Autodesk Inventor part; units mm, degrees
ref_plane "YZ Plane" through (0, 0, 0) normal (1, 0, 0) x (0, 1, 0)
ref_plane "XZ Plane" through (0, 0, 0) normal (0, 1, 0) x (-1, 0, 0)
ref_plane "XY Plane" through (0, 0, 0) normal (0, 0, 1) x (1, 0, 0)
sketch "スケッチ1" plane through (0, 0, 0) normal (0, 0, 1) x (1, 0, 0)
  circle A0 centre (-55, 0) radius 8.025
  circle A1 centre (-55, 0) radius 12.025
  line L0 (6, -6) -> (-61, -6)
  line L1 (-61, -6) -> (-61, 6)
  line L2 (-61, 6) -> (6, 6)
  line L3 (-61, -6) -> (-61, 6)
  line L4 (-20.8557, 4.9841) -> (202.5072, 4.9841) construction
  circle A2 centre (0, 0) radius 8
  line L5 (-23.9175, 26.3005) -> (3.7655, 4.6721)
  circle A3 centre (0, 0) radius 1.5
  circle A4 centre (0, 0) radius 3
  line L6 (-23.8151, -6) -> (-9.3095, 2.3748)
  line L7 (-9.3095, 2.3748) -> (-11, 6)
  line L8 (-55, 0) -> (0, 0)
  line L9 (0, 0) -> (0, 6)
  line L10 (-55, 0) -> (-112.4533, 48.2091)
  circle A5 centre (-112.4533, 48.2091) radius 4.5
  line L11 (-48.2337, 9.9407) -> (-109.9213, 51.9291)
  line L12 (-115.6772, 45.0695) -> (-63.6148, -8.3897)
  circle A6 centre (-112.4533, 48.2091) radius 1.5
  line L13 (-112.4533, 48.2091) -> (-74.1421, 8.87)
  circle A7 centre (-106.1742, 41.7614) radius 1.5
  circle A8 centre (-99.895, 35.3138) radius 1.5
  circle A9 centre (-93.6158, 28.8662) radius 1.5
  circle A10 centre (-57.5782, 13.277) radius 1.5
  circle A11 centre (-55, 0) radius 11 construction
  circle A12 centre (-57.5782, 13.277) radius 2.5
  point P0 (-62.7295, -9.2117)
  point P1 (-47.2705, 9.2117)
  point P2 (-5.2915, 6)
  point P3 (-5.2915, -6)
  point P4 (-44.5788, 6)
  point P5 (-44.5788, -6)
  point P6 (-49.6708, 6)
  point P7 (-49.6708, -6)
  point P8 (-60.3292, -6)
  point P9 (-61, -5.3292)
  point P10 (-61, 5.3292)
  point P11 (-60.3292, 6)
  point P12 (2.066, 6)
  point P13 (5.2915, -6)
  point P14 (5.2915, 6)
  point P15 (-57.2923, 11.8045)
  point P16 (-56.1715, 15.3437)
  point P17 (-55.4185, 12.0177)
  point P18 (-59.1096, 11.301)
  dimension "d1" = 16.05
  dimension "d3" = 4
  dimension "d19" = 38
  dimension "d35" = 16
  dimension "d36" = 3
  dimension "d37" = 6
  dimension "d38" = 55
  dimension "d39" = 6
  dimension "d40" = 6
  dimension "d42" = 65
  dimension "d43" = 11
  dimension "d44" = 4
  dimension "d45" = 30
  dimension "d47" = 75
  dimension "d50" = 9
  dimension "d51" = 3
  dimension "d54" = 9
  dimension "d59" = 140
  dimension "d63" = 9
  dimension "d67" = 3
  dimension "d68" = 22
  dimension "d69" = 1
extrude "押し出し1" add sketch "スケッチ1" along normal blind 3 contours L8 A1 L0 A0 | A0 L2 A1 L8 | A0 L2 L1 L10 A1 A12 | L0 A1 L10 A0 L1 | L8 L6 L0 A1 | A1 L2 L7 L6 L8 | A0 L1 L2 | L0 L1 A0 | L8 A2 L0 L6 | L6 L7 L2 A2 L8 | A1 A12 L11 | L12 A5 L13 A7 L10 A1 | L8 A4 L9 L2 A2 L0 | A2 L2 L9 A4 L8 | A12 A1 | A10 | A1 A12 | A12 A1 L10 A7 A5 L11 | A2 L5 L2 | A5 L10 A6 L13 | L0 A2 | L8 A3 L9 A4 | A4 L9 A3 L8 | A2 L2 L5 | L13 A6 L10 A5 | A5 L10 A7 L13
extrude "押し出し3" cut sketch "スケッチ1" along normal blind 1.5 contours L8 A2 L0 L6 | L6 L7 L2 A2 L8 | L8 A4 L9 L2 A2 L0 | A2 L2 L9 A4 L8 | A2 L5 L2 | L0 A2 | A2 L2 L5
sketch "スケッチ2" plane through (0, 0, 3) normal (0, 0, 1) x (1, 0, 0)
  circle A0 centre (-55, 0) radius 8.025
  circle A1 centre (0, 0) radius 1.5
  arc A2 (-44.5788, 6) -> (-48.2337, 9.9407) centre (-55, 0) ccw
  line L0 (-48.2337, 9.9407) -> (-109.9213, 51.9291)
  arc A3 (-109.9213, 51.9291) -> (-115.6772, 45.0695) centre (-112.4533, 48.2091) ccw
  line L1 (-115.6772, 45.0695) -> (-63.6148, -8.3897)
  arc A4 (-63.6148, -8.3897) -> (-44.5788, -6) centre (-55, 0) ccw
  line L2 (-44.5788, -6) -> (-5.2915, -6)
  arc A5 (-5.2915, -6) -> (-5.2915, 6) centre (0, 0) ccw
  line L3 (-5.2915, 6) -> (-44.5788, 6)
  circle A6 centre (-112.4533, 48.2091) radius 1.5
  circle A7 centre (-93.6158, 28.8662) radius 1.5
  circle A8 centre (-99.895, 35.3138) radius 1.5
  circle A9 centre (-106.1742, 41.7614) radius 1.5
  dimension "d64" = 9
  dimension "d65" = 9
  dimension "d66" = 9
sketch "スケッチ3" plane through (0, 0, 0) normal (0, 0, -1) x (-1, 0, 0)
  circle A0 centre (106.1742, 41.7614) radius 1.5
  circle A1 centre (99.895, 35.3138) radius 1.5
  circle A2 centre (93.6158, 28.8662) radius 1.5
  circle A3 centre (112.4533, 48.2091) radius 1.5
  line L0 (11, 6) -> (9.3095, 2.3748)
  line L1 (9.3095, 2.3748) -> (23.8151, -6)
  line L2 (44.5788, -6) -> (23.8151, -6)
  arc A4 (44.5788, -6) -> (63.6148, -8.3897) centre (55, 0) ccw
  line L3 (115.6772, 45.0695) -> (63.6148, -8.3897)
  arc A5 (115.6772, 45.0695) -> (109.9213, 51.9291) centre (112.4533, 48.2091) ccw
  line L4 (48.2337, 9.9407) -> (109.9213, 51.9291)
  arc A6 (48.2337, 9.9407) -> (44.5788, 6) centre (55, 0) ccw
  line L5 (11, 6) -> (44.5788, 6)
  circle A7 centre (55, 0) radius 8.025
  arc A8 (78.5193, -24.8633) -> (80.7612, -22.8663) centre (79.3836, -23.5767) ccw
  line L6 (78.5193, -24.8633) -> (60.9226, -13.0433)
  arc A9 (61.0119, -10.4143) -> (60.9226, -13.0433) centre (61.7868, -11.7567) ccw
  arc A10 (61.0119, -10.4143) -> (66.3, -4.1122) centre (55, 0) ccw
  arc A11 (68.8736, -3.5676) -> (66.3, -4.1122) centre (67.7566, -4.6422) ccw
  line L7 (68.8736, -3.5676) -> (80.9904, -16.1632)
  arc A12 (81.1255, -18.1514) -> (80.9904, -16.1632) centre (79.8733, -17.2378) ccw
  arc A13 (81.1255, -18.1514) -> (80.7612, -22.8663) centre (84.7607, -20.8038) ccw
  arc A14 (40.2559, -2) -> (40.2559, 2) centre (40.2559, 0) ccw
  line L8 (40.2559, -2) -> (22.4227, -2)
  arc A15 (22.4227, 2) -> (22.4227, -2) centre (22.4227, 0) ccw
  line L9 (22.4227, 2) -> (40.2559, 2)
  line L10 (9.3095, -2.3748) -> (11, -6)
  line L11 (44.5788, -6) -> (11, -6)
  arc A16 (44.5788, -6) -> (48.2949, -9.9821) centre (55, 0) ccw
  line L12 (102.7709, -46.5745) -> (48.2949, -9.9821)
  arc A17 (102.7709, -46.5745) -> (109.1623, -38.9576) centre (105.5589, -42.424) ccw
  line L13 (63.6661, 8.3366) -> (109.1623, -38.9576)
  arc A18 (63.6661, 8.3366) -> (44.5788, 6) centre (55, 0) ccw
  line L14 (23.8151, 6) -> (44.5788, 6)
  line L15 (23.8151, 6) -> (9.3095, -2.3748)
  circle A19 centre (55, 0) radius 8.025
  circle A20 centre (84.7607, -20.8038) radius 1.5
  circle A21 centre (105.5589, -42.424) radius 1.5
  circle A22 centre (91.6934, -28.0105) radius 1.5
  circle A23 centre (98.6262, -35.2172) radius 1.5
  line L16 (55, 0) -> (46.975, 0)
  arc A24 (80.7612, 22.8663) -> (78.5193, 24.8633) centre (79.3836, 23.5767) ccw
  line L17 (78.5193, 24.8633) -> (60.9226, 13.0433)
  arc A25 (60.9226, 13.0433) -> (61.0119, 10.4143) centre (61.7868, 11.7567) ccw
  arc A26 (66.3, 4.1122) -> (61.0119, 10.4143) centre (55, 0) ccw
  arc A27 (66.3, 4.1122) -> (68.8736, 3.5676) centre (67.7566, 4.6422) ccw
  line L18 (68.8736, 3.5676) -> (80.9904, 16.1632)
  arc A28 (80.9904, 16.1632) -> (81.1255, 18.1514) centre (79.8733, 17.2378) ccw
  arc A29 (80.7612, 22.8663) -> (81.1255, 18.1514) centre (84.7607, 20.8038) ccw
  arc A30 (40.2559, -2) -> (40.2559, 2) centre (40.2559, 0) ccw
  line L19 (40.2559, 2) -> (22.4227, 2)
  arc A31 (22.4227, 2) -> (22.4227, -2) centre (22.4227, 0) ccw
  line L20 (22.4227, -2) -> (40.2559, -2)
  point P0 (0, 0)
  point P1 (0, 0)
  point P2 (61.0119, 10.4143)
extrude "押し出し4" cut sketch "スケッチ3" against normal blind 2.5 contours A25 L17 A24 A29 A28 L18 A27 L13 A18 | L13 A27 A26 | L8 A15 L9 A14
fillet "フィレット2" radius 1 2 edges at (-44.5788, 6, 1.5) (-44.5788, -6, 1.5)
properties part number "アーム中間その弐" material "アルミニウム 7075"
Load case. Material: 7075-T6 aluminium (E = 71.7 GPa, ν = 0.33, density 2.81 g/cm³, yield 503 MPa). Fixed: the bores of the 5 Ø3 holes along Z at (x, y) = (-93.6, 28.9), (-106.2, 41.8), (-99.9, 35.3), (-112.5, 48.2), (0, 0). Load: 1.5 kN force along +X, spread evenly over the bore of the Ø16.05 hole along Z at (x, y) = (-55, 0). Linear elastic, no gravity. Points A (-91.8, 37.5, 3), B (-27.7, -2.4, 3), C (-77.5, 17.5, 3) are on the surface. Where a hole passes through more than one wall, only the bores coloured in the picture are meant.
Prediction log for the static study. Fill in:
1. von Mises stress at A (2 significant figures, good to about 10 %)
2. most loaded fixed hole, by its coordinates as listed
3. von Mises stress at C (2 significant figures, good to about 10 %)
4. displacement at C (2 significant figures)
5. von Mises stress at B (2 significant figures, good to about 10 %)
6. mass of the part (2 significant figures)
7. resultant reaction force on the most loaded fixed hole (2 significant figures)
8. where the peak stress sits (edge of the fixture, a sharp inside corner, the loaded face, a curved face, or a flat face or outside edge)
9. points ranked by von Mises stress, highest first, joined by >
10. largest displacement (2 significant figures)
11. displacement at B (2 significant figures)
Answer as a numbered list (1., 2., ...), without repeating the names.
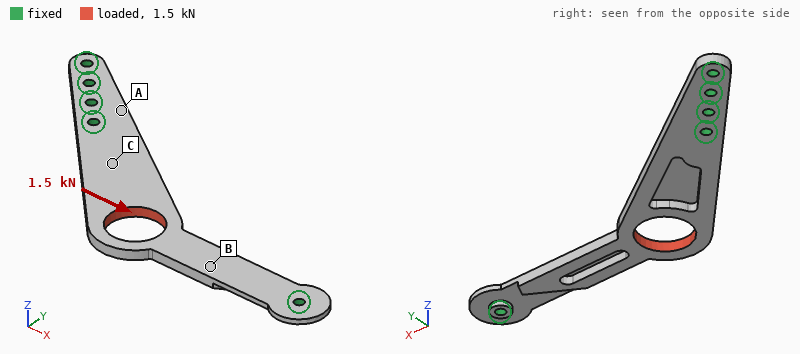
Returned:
1. 19 MPa
2. (0, 0)
3. 43 MPa
4. 0.046 mm
5. 71 MPa
6. 13 g
7. 1.1 kN
8. a curved face
9. B > C > A
10. 0.20 mm
11. 0.11 mm
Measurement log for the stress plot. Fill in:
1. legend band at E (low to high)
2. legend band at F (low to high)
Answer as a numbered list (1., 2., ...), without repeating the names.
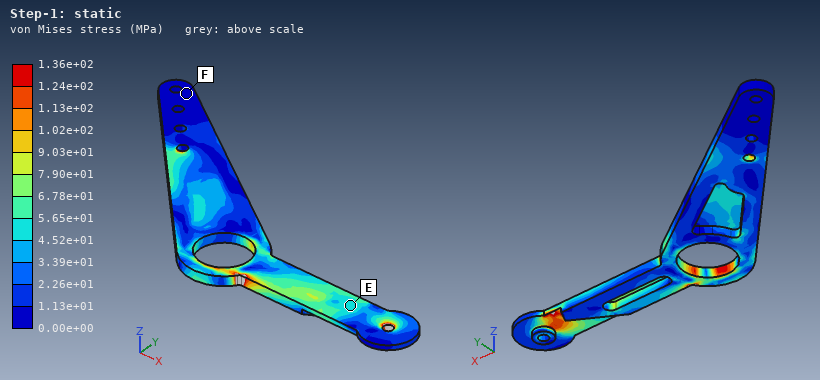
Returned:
1. 4.52e+01 to 5.65e+01 MPa
2. 0.00e+00 to 1.13e+01 MPa
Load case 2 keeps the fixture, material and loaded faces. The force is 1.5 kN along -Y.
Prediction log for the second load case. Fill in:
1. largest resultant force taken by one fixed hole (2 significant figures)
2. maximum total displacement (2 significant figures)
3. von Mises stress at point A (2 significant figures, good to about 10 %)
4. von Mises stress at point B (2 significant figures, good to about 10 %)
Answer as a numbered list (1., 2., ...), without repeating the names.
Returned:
1. 1.3 kN
2. 0.31 mm
3. 68 MPa
4. 77 MPa
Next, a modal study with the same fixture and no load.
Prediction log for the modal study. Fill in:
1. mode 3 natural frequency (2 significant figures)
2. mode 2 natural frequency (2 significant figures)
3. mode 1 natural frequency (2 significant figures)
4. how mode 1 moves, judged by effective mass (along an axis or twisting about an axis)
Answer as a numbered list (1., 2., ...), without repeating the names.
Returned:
1. 3800 Hz
2. 3100 Hz
3. 1100 Hz
4. along Z
